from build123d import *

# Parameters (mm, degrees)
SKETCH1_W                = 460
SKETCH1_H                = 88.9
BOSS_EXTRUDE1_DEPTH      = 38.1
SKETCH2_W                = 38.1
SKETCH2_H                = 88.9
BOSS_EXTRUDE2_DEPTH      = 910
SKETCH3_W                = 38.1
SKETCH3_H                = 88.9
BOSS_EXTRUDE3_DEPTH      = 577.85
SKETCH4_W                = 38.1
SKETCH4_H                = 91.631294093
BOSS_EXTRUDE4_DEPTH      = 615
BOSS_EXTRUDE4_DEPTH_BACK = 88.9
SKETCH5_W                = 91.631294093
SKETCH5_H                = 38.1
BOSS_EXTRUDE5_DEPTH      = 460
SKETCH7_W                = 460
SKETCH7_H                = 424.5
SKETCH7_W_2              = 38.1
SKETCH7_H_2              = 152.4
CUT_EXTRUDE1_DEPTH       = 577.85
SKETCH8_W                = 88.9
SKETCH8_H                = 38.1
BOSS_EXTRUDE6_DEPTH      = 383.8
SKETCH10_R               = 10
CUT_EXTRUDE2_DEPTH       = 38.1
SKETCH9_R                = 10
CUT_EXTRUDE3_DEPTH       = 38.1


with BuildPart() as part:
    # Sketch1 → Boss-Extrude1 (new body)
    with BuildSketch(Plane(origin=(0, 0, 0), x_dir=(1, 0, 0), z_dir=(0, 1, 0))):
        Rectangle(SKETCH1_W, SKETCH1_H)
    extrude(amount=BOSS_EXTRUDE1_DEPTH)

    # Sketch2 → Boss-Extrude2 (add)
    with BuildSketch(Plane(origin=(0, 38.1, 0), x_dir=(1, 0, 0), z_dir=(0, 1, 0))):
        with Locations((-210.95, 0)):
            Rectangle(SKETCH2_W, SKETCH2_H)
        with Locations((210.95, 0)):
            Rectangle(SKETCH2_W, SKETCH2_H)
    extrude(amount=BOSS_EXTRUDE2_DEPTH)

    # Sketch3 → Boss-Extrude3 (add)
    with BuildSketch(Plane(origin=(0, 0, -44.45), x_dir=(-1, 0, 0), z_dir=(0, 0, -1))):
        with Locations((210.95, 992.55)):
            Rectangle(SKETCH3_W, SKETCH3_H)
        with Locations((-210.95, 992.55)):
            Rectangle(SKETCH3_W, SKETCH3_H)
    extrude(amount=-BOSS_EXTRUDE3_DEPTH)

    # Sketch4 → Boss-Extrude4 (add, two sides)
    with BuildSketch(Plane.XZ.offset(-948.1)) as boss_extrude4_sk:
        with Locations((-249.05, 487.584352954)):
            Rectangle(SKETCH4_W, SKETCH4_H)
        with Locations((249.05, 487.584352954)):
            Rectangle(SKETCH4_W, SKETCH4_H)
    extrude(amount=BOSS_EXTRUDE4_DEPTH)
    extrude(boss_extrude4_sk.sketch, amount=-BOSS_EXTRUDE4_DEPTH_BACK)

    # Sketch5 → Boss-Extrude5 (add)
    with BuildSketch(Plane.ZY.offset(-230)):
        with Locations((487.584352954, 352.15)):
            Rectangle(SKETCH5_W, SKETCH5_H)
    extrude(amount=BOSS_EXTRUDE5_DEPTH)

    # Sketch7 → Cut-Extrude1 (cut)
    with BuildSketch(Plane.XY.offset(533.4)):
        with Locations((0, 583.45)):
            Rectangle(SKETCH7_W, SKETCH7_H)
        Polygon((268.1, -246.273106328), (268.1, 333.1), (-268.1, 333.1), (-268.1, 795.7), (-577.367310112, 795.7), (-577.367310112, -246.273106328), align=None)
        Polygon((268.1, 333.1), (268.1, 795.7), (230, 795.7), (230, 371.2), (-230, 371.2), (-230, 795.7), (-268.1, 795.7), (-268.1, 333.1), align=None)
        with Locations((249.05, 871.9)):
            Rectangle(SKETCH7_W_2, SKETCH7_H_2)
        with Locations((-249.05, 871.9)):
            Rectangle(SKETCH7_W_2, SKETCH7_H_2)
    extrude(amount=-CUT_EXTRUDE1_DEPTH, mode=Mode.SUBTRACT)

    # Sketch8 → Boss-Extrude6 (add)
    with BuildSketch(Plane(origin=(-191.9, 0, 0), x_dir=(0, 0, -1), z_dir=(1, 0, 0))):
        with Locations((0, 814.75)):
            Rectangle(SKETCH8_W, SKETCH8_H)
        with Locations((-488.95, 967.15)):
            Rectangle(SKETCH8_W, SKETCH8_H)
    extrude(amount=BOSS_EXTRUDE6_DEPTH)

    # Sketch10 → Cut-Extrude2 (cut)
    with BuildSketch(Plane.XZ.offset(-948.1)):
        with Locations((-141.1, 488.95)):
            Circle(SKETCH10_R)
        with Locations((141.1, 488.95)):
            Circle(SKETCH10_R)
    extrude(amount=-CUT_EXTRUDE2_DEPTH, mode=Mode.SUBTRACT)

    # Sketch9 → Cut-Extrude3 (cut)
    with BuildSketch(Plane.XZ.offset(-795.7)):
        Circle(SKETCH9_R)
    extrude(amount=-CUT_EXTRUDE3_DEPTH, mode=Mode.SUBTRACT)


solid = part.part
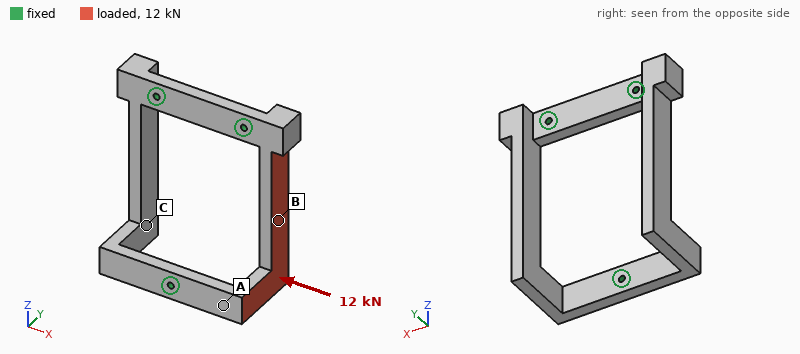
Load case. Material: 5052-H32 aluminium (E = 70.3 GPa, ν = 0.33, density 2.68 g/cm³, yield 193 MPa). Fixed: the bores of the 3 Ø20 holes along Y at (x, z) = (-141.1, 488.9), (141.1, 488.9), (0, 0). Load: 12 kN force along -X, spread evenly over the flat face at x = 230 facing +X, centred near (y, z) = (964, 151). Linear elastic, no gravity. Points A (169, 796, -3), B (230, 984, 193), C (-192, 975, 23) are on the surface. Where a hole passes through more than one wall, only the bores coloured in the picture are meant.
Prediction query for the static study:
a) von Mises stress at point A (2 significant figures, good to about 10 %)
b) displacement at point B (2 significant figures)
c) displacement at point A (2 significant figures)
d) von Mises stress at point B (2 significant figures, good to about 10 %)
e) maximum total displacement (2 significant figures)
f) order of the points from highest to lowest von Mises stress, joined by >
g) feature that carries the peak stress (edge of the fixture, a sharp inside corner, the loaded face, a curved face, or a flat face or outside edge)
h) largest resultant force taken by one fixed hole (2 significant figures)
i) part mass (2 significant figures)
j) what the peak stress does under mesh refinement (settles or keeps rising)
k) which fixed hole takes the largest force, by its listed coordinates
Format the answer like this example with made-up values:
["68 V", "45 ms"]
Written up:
["22 MPa", "0.59 mm", "0.23 mm", "16 MPa", "1.1 mm", "A > B > C", "edge of the fixture", "7.0 kN", "22 kg", "keeps rising", "(0, 0)"]
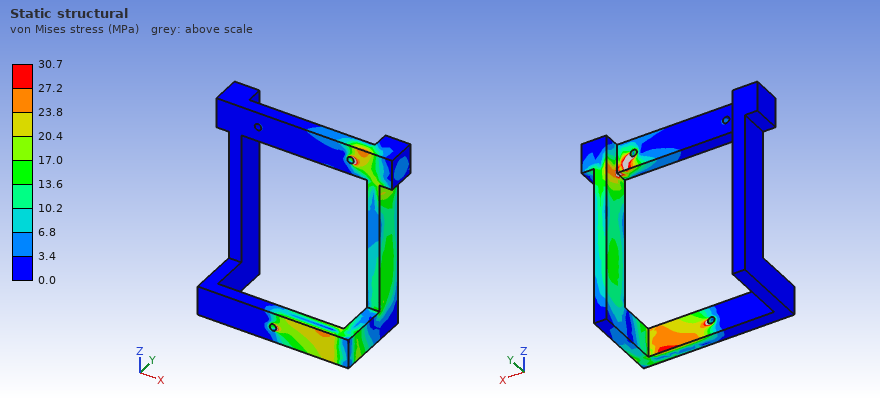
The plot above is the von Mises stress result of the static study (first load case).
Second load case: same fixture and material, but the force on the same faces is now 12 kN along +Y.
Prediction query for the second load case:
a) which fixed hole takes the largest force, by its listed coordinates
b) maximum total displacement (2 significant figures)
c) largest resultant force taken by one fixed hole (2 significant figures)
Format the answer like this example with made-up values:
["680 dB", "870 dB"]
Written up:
["(0, 0)", "1.1 mm", "6.7 kN"]
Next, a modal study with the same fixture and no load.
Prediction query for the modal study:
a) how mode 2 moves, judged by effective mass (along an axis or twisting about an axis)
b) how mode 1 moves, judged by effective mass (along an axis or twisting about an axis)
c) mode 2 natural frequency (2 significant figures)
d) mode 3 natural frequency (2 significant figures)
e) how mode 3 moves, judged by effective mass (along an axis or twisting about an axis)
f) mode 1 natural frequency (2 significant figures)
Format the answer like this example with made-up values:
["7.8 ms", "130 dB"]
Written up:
["along Y", "along X", "250 Hz", "470 Hz", "along X", "240 Hz"]
